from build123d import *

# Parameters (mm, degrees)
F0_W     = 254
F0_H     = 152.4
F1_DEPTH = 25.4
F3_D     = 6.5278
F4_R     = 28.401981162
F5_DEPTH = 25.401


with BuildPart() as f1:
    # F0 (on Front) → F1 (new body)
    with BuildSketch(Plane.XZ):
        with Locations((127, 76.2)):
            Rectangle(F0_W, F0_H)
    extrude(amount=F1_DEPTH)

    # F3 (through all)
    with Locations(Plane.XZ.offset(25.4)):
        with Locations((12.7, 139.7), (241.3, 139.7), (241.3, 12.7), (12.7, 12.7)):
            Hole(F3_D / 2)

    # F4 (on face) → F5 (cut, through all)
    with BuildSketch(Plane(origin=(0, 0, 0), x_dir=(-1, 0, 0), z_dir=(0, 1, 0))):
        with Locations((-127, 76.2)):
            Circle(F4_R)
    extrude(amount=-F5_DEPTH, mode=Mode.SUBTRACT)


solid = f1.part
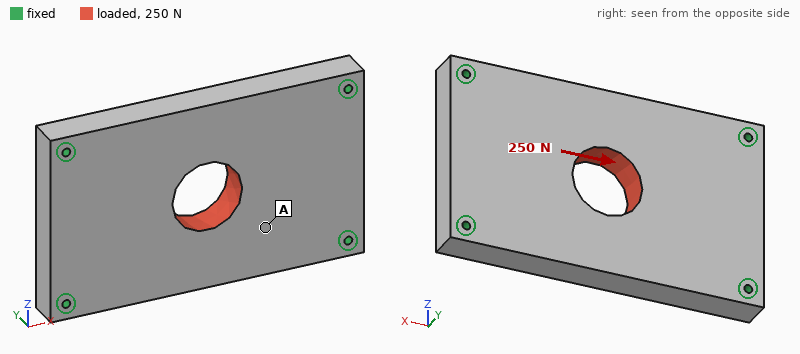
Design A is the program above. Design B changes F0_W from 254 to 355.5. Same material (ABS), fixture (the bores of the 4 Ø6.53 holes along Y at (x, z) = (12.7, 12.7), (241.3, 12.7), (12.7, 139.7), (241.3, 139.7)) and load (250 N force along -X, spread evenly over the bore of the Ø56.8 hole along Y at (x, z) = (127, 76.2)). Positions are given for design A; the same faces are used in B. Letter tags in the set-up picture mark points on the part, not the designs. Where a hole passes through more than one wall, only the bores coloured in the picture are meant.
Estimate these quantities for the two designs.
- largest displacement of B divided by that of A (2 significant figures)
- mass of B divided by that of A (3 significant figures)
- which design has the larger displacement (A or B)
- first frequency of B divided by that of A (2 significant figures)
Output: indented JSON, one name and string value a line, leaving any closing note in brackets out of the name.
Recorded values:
{
  "largest displacement of B divided by that of A": "0.88",
  "mass of B divided by that of A": "1.43",
  "which design has the larger displacement": "A",
  "first frequency of B divided by that of A": "1.0"
}
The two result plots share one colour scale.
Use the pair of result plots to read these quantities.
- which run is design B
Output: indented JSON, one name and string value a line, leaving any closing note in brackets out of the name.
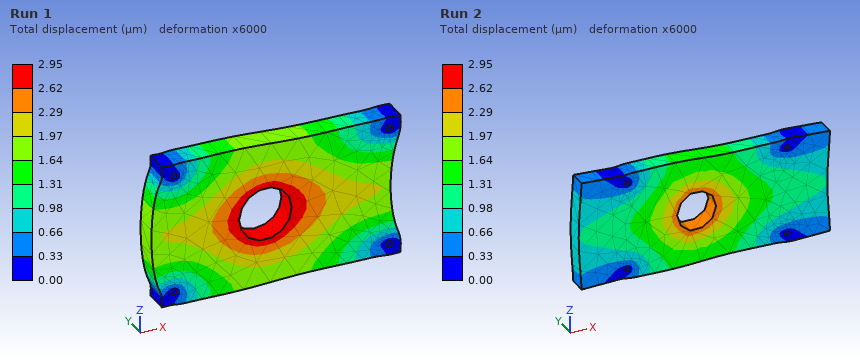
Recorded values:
{
  "which run is design B": "Run 2"
}
